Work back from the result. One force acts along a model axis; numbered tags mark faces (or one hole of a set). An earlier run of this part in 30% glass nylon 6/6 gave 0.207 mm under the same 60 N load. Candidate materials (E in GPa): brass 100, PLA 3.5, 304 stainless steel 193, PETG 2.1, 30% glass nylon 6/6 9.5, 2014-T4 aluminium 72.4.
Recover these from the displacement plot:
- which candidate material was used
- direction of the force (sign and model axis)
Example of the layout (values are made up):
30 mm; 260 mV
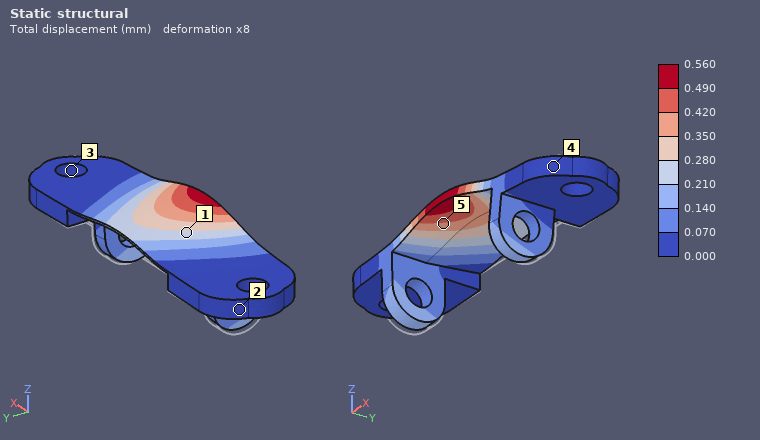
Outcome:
PLA; +Z
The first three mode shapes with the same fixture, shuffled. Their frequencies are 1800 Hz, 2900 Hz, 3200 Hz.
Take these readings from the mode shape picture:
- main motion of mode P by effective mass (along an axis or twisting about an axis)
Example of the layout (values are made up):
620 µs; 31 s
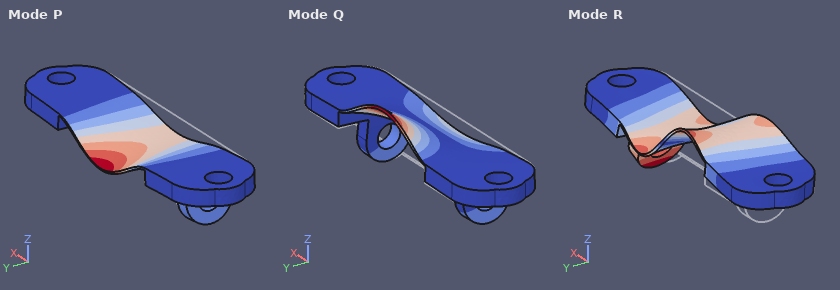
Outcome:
along Z
